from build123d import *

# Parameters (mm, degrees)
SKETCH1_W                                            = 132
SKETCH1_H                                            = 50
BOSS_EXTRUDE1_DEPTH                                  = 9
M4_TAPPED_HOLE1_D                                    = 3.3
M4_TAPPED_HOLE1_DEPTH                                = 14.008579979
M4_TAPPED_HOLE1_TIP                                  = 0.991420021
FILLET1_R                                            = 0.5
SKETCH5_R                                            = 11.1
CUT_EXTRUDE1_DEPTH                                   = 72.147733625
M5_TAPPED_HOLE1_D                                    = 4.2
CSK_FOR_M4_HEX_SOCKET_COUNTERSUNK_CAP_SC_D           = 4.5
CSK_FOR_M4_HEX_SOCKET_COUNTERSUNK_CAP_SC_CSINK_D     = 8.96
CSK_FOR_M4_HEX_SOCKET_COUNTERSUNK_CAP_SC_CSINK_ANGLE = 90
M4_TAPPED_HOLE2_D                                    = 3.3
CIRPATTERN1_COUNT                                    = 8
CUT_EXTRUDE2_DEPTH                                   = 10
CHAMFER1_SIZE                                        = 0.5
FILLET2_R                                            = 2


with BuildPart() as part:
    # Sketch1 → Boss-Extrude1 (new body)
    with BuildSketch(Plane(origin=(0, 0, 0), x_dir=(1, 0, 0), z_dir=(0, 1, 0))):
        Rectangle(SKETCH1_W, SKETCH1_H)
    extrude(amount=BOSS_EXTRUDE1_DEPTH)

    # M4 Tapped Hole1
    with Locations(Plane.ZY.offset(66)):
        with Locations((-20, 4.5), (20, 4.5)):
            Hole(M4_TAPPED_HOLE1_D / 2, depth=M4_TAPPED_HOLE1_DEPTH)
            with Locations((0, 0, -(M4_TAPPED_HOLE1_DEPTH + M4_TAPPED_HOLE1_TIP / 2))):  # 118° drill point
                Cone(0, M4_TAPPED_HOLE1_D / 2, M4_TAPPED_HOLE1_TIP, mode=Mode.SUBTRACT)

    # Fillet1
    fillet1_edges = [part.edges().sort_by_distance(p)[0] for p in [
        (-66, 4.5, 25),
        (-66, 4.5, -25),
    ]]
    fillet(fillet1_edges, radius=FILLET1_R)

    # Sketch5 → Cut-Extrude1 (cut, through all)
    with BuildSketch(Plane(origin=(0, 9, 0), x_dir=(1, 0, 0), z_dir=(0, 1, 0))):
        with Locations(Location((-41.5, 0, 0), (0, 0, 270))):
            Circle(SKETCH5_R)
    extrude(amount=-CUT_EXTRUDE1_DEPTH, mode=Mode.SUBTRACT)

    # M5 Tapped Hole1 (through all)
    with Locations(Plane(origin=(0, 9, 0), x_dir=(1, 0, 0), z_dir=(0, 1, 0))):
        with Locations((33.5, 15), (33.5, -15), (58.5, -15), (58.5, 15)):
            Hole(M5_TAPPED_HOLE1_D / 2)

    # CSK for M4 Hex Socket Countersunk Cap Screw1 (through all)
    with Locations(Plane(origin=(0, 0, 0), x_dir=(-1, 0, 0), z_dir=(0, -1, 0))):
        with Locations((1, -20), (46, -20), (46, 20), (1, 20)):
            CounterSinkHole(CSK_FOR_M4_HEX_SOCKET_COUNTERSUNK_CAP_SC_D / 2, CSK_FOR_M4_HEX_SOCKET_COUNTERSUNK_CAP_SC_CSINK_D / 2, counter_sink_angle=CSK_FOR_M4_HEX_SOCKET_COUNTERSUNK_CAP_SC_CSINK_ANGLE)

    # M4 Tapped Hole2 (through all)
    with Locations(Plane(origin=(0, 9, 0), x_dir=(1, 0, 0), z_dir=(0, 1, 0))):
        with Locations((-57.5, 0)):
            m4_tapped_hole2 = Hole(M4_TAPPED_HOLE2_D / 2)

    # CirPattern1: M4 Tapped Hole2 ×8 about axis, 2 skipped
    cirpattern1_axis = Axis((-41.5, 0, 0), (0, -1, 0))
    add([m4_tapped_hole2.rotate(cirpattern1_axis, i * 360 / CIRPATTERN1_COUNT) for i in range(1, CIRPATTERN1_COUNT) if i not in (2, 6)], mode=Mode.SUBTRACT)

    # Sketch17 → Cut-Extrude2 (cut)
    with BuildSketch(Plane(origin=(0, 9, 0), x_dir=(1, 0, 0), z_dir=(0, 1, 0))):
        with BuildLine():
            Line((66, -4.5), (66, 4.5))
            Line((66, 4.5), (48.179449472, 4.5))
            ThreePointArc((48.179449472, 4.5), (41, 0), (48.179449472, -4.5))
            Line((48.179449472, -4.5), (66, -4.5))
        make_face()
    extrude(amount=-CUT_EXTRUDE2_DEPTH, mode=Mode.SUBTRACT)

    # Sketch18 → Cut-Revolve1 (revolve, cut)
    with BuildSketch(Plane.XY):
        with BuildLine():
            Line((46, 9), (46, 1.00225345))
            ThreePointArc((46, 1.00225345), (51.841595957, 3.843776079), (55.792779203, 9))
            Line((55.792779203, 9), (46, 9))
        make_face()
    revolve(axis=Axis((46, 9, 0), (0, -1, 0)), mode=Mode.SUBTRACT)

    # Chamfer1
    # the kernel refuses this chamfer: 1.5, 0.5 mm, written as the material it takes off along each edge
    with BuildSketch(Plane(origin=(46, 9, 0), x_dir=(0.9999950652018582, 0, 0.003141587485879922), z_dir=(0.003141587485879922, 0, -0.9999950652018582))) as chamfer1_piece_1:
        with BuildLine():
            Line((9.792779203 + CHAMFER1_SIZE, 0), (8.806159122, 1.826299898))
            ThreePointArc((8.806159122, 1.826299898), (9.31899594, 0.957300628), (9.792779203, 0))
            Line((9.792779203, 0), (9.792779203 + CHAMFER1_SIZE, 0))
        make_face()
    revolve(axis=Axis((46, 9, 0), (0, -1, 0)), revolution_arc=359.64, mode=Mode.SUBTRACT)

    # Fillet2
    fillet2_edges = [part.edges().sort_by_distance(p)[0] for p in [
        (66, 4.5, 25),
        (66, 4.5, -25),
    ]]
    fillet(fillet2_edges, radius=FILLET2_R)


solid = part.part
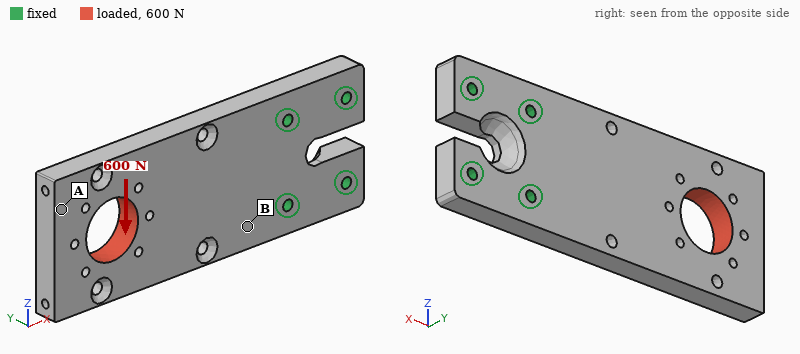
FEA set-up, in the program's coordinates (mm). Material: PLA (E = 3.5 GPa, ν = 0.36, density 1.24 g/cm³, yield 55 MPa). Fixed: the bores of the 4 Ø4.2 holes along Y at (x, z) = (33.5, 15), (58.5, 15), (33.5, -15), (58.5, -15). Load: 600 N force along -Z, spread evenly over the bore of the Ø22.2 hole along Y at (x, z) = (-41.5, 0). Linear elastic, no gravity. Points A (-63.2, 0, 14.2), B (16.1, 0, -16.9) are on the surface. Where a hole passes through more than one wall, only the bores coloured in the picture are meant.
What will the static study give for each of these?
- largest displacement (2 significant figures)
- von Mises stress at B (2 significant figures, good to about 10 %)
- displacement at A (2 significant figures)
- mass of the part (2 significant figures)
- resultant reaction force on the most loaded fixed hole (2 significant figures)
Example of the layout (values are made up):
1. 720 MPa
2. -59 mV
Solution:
1. 0.64 mm
2. 6.7 MPa
3. 0.60 mm
4. 64 g
5. 1.2 kN
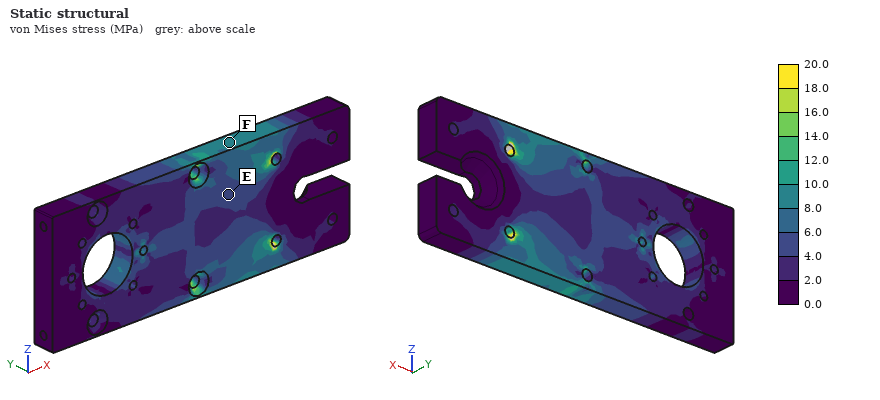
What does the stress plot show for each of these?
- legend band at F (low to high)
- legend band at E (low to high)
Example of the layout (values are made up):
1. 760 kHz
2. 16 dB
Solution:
1. 8.0 to 10.0 MPa
2. 4.0 to 6.0 MPa
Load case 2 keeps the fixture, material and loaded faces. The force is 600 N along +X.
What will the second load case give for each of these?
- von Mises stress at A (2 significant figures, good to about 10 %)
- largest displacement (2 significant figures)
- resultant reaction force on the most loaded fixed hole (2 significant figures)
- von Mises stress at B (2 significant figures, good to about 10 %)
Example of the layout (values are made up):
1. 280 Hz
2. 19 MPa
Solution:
1. 0.59 MPa
2. 52 µm
3. 260 N
4. 1.4 MPa
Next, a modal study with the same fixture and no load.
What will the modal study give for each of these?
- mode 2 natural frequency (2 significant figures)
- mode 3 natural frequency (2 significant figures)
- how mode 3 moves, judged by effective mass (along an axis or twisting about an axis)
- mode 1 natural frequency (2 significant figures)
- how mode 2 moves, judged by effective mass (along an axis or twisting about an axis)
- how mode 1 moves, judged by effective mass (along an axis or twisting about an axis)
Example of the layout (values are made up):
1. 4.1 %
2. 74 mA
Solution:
1. 940 Hz
2. 1100 Hz
3. along Z
4. 260 Hz
5. twisting about X
6. along Y
